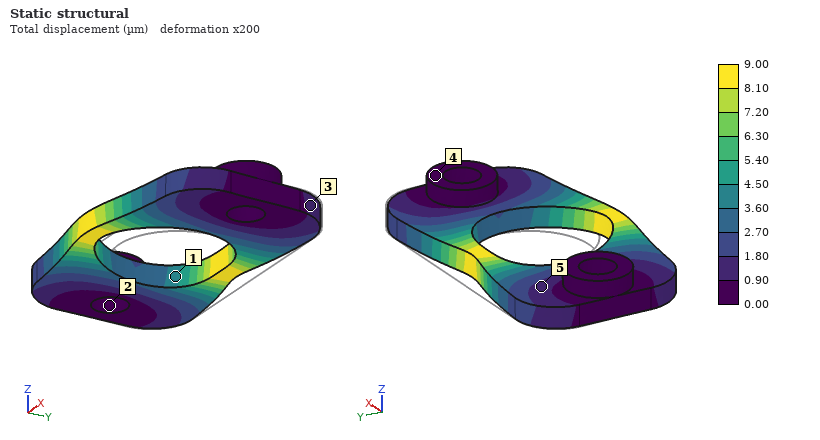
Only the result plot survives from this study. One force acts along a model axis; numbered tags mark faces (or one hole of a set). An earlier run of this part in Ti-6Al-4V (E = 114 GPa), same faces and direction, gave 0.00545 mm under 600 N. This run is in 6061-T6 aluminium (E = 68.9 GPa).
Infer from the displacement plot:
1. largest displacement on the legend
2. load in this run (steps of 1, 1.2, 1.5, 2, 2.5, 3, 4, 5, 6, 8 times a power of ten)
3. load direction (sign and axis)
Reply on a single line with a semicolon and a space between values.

9.00 µm; 600 N; -Y
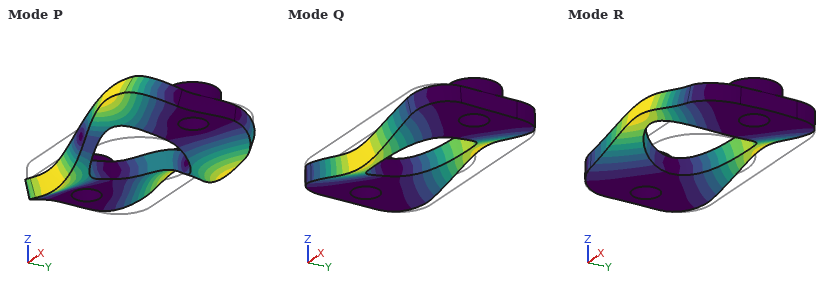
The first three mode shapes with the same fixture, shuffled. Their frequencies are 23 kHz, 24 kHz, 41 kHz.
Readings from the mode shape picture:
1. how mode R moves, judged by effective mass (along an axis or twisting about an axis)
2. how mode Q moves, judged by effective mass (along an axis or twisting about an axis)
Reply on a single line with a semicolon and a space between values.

along Z; twisting about X
